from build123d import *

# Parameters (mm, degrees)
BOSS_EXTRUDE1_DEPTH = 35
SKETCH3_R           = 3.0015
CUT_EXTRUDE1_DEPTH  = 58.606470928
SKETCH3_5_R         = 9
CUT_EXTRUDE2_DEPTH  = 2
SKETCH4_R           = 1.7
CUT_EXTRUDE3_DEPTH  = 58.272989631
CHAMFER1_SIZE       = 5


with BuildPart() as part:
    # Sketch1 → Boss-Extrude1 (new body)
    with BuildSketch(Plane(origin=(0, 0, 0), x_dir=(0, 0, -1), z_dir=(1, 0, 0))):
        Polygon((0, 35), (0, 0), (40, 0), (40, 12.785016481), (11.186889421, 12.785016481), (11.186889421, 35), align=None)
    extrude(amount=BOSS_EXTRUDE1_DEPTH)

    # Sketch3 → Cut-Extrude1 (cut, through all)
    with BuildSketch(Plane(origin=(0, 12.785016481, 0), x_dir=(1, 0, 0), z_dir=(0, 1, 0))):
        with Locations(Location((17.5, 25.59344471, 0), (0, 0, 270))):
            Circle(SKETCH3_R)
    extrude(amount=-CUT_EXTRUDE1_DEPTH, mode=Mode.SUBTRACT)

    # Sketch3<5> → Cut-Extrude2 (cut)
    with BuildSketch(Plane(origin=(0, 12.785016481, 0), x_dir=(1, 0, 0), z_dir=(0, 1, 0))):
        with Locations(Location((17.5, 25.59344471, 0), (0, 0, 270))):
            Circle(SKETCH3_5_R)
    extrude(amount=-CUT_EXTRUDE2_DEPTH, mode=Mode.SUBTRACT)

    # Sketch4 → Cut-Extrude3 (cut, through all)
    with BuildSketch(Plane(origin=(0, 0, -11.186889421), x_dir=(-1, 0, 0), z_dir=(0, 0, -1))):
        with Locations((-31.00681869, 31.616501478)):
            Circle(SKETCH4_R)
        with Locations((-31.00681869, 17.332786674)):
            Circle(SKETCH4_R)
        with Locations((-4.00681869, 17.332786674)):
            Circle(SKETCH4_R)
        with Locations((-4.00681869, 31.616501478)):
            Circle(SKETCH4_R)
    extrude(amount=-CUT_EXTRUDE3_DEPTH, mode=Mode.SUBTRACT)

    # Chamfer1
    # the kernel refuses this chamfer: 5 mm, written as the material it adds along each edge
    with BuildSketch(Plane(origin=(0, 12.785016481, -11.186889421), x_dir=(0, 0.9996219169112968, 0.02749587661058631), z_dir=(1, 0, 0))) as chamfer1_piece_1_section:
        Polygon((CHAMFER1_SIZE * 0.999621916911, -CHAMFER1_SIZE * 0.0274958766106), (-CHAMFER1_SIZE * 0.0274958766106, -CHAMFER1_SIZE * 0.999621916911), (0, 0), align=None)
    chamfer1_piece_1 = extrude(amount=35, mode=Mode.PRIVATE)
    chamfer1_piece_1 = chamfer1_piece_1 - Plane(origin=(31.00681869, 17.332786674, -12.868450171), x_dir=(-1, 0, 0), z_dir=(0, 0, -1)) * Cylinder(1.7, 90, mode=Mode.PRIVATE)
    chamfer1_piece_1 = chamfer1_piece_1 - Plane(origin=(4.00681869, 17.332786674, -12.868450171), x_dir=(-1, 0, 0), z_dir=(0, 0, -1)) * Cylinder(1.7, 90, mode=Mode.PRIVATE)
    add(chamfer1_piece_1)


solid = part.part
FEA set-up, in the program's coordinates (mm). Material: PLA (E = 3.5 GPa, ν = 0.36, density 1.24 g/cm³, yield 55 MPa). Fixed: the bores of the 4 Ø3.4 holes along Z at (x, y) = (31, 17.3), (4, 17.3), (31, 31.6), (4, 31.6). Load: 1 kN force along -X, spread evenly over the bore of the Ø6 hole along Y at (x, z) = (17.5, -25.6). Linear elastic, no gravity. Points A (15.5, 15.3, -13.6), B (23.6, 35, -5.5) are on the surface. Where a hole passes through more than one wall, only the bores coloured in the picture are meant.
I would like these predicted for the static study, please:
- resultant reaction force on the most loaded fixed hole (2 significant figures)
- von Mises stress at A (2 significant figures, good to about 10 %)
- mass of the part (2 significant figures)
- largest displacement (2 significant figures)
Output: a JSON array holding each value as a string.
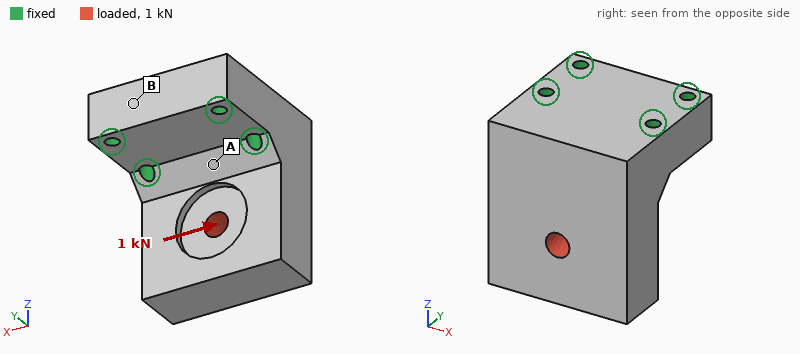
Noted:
["850 N", "8.6 MPa", "32 g", "0.16 mm"]
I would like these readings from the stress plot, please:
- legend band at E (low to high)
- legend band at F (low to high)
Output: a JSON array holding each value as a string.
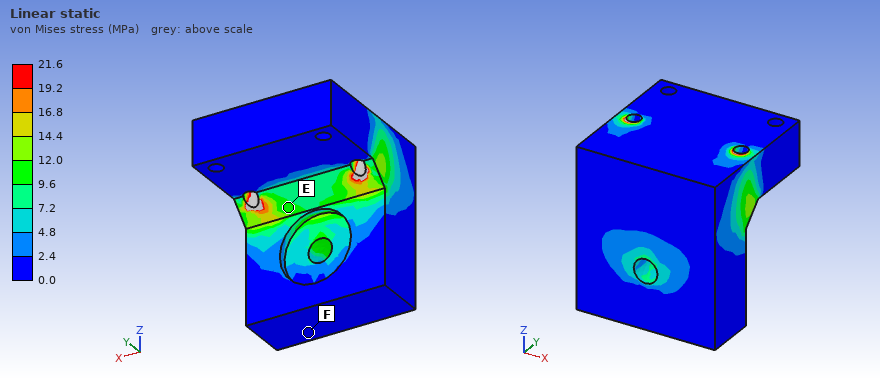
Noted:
["9.6 to 12.0 MPa", "0.0 to 2.4 MPa"]
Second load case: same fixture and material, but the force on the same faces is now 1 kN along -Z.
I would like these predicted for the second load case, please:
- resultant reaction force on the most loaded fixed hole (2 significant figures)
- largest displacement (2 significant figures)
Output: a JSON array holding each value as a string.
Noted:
["560 N", "0.21 mm"]
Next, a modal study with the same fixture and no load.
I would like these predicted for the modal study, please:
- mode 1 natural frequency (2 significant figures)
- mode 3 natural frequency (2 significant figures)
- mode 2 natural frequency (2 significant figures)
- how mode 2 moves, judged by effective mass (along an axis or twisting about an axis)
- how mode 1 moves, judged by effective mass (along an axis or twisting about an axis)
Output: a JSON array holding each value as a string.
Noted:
["2200 Hz", "5400 Hz", "3600 Hz", "along X", "along Y"]
